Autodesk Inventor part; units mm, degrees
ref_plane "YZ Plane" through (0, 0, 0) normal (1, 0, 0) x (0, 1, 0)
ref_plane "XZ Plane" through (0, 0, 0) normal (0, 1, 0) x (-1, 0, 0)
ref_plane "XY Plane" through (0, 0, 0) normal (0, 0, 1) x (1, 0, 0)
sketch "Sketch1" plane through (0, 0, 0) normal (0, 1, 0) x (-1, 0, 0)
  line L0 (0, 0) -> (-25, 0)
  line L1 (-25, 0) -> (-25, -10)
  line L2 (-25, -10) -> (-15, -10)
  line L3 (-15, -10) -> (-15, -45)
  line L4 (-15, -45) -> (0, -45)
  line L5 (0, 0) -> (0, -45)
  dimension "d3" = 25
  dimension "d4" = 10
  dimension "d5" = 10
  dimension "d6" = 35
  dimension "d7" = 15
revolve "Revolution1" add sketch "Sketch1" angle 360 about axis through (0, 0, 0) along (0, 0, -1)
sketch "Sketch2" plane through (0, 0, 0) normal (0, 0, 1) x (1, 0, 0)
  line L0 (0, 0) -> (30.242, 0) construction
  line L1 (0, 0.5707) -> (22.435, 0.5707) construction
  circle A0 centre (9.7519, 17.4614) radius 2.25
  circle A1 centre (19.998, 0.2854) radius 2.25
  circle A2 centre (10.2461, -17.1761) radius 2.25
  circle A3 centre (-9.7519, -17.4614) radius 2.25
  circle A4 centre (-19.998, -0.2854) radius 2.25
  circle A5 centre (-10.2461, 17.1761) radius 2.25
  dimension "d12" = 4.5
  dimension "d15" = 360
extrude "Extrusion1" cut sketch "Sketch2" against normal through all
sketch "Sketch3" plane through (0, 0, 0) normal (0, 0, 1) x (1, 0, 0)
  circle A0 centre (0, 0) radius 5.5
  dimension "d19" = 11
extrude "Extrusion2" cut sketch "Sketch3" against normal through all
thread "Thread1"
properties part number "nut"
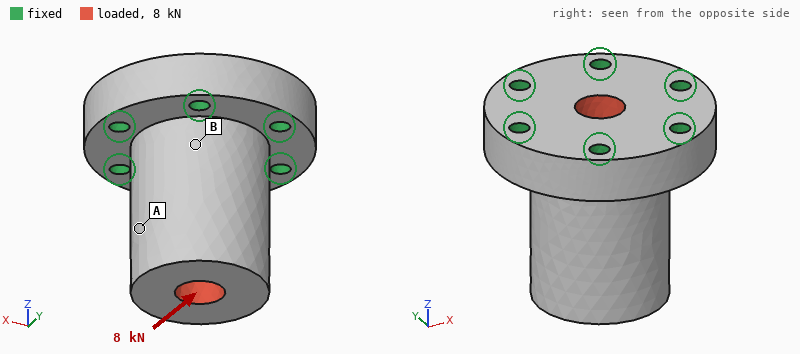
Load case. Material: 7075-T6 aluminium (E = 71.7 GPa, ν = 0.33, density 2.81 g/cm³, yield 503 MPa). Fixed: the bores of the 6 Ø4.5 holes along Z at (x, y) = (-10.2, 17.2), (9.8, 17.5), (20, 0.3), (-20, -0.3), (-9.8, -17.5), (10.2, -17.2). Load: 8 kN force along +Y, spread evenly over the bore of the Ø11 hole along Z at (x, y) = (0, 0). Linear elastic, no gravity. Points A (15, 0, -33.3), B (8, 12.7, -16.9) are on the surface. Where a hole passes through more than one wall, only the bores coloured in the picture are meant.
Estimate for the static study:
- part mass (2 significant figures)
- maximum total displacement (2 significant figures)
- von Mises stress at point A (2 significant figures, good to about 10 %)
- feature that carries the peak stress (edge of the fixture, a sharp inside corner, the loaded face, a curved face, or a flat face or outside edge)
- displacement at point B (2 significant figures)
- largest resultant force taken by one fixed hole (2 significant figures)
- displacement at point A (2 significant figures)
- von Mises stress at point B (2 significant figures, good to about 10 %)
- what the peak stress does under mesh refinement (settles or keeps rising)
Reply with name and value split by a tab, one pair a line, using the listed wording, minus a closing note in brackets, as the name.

part mass	110 g
maximum total displacement	38 µm
von Mises stress at point A	8.1 MPa
feature that carries the peak stress	edge of the fixture
displacement at point B	12 µm
largest resultant force taken by one fixed hole	2.8 kN
displacement at point A	24 µm
von Mises stress at point B	24 MPa
what the peak stress does under mesh refinement	keeps rising
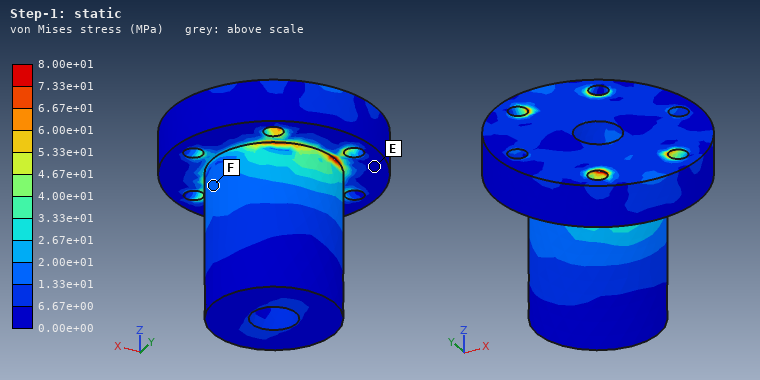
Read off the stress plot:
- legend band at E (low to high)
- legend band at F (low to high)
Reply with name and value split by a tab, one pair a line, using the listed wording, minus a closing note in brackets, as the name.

legend band at E	0.00e+00 to 6.67e+00 MPa
legend band at F	1.33e+01 to 2.00e+01 MPa
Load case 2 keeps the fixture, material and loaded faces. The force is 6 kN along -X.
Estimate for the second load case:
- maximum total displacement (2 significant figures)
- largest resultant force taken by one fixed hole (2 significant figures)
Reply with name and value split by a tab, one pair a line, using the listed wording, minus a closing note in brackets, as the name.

maximum total displacement	28 µm
largest resultant force taken by one fixed hole	2.4 kN
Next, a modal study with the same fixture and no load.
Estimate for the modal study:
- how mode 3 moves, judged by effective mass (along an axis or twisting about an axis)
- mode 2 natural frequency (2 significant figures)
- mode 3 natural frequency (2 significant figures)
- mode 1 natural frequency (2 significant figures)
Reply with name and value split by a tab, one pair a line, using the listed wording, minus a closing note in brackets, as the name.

how mode 3 moves, judged by effective mass	twisting about Z
mode 2 natural frequency	10000 Hz
mode 3 natural frequency	20 kHz
mode 1 natural frequency	9900 Hz
